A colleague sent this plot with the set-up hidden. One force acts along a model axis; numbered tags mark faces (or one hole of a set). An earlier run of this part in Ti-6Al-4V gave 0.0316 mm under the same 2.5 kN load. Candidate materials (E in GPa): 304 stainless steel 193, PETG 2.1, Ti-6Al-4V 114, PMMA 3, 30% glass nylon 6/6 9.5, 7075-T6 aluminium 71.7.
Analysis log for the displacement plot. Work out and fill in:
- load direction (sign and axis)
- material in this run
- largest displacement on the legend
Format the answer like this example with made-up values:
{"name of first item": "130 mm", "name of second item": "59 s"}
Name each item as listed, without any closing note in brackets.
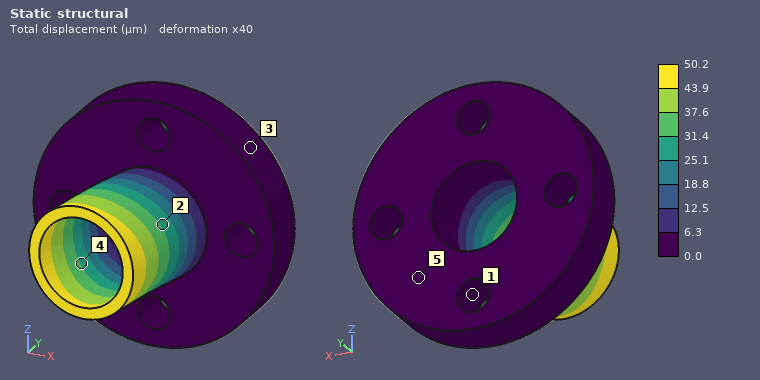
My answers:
{"load direction": "-X", "material in this run": "7075-T6 aluminium", "largest displacement on the legend": "50.2 µm"}
